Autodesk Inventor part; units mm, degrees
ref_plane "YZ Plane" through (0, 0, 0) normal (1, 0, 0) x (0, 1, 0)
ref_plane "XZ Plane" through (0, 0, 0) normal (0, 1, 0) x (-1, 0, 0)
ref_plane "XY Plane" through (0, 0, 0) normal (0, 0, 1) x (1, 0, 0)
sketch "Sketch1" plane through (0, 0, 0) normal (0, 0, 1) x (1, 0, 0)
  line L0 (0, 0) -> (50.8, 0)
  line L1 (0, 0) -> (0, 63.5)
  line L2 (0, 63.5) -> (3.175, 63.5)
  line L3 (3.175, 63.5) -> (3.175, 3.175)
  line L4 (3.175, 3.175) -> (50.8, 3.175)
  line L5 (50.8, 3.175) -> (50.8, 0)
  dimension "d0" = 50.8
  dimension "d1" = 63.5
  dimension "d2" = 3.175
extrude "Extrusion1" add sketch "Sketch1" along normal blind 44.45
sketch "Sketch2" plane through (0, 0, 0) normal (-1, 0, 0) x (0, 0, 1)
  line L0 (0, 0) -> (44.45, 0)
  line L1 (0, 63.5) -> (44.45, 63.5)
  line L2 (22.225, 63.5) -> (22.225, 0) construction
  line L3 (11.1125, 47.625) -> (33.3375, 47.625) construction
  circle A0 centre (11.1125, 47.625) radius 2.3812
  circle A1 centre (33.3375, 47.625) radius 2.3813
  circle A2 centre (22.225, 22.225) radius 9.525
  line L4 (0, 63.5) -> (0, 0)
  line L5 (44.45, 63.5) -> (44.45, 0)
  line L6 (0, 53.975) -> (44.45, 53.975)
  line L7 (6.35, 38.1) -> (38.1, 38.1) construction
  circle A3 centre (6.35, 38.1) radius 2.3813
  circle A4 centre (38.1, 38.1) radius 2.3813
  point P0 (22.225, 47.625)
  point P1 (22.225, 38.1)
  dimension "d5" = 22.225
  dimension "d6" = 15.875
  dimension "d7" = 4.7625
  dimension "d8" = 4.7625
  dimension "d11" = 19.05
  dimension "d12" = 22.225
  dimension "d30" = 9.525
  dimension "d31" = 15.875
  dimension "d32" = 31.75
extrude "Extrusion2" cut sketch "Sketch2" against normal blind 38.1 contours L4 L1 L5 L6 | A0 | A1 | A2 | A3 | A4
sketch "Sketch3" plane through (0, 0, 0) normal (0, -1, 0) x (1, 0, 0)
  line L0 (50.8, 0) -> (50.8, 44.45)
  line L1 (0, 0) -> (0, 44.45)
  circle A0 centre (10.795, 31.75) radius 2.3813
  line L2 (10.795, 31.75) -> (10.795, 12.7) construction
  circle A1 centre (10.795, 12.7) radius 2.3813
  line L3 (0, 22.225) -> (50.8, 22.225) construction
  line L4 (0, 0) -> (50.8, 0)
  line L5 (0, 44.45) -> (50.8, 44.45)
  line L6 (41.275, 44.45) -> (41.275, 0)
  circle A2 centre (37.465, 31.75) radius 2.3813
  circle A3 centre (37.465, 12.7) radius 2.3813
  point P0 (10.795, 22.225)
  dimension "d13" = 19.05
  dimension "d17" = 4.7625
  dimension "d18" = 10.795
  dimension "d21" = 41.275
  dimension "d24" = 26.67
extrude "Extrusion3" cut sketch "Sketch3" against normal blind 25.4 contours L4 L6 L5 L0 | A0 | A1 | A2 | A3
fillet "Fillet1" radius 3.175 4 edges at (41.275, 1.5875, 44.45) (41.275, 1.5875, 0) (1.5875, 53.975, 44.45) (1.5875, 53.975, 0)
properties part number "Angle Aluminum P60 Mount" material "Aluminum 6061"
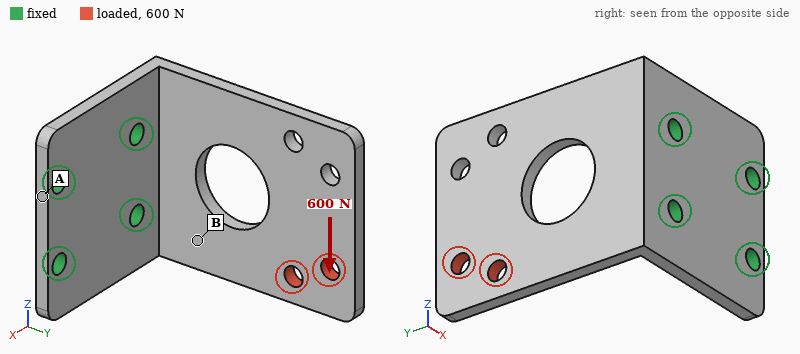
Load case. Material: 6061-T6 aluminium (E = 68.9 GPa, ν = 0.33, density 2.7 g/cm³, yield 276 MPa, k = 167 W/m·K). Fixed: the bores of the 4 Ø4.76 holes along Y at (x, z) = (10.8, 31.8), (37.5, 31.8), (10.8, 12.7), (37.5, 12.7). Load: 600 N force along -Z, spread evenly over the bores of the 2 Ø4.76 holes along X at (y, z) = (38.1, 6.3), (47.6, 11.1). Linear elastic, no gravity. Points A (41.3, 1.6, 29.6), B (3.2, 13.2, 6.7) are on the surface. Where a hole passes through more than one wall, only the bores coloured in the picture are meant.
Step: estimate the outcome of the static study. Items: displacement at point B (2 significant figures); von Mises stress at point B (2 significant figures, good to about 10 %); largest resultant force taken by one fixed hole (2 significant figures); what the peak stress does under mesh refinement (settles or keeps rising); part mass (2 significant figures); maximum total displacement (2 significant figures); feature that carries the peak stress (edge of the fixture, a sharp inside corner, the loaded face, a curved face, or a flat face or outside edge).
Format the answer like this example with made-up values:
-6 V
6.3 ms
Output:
0.090 mm
42 MPa
1.1 kN
keeps rising
31 g
0.27 mm
edge of the fixture
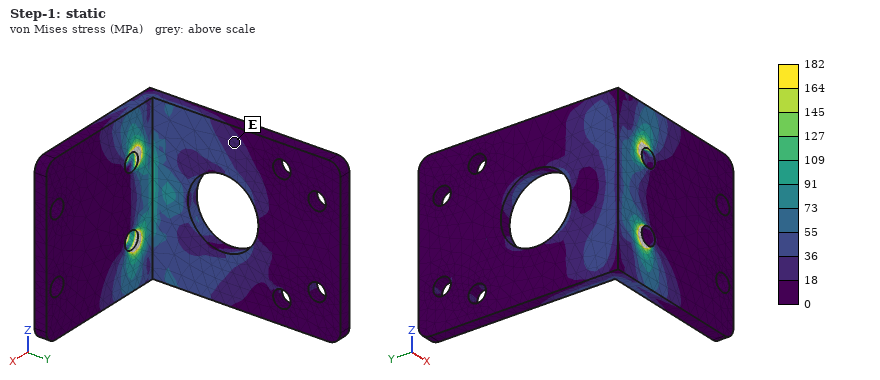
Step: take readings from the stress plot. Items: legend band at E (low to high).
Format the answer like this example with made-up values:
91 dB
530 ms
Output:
18 to 36 MPa
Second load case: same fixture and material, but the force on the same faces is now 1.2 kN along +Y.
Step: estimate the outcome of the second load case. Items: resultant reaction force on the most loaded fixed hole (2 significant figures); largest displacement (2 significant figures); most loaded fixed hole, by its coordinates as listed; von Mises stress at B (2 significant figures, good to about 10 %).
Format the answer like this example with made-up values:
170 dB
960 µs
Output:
1.3 kN
0.39 mm
(10.8, 12.7)
40 MPa
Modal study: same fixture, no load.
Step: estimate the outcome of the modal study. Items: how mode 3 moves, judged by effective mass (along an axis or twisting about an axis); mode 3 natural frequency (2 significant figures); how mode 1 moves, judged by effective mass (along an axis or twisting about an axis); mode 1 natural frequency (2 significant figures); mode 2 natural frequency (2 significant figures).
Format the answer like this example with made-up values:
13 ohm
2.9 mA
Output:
along Z
3000 Hz
along X
740 Hz
2100 Hz
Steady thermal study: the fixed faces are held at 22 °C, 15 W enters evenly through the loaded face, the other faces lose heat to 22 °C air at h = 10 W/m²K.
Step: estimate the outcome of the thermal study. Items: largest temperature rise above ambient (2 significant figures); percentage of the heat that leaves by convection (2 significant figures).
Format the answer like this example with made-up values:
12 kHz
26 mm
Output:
49 K
8.4 %
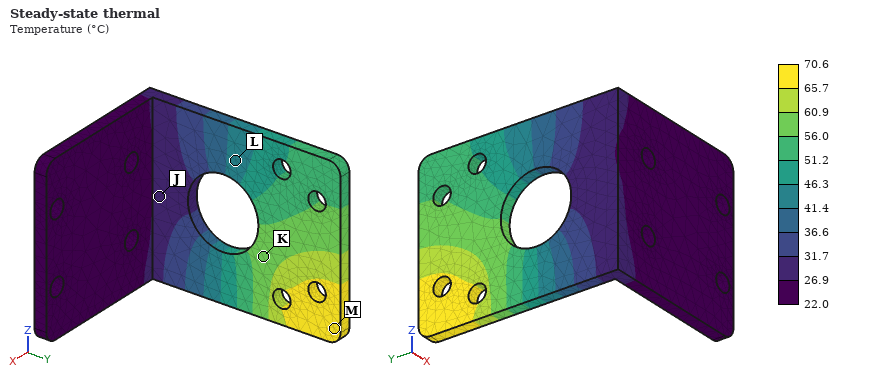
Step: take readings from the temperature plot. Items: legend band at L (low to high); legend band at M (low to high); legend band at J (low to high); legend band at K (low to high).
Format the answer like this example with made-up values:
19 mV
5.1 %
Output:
41.4 to 46.3 °C
65.7 to 70.6 °C
26.9 to 31.7 °C
56.0 to 60.9 °C
